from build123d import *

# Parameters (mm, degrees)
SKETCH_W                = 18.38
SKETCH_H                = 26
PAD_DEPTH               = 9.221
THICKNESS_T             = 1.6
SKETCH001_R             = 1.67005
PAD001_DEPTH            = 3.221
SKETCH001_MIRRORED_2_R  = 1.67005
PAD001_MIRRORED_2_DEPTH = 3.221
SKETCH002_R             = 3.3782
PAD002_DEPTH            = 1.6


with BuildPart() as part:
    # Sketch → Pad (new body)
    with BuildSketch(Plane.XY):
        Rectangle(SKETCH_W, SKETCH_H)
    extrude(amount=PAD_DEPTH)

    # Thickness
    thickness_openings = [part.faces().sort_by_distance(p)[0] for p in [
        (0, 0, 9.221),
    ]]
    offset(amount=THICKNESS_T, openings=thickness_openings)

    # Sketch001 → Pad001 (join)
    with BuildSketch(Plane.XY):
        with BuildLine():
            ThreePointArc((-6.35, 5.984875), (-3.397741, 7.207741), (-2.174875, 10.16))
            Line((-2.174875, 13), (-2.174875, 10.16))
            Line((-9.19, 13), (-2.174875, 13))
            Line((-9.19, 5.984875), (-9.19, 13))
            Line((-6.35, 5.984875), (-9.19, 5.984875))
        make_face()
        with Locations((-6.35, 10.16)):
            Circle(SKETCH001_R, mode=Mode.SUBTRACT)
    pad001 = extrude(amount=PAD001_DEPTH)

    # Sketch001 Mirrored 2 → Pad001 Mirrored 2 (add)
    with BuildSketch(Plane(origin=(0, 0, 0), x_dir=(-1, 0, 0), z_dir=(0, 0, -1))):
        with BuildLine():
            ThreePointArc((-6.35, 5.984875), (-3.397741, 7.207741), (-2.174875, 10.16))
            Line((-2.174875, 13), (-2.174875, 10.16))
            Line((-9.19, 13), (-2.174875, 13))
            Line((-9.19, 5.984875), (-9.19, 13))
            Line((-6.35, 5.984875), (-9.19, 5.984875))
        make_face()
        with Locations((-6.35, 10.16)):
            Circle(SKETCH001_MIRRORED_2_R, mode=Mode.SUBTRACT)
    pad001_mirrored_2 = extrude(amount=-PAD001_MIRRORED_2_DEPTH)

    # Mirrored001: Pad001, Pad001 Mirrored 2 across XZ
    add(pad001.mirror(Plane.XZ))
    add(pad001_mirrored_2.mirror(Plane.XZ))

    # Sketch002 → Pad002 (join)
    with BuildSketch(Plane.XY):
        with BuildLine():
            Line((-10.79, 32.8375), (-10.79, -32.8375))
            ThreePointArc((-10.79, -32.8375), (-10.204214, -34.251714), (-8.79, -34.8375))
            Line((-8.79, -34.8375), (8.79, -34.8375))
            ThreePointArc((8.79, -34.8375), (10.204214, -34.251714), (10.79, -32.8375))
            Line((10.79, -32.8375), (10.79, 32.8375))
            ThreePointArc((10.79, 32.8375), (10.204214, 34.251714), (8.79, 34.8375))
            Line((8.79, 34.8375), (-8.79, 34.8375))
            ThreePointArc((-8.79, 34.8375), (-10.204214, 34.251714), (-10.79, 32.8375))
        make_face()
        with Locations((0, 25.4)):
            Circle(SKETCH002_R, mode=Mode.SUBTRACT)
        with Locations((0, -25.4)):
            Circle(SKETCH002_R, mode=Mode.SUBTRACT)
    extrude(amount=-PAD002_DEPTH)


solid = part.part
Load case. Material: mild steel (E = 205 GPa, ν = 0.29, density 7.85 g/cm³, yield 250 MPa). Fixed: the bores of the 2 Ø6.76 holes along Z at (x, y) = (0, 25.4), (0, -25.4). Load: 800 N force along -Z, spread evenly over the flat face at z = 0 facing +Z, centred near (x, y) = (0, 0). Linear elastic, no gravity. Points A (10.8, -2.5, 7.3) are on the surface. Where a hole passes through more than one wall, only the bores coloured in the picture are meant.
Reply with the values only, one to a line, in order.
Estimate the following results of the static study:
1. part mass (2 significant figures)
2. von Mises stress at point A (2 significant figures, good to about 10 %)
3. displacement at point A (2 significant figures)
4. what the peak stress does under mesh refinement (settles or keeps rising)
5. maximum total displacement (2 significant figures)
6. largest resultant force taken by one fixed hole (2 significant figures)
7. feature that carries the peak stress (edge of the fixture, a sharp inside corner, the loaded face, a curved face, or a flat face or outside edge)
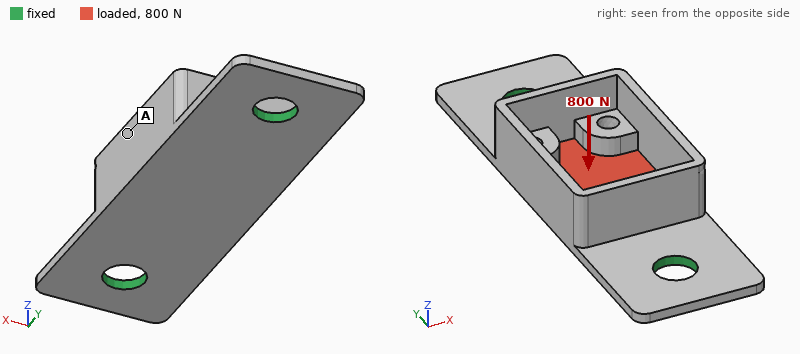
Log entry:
33 g
46 MPa
31 µm
keeps rising
39 µm
540 N
edge of the fixture
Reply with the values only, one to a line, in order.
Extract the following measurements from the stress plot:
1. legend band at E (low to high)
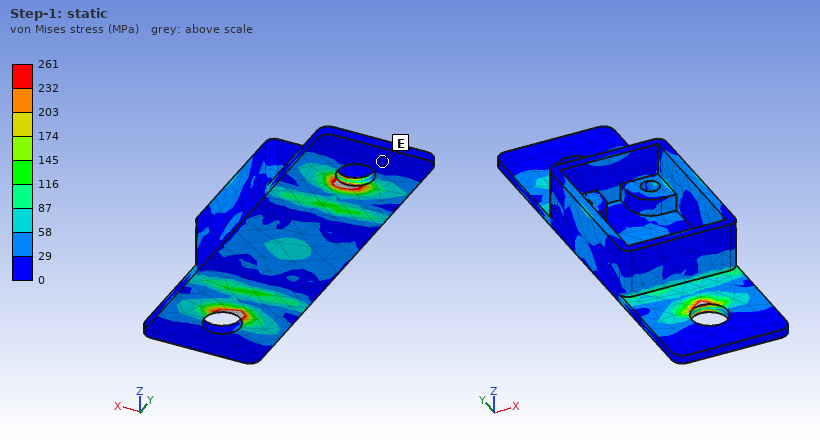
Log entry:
0 to 29 MPa
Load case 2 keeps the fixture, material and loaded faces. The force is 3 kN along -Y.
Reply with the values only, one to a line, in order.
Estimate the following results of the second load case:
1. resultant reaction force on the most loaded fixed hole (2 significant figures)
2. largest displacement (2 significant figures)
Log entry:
1.5 kN
5.2 µm
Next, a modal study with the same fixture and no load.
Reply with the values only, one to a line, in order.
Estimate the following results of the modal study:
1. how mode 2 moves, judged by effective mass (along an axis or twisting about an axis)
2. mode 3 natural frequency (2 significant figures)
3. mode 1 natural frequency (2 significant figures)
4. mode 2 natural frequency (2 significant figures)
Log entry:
along Z
9700 Hz
3700 Hz
5500 Hz
